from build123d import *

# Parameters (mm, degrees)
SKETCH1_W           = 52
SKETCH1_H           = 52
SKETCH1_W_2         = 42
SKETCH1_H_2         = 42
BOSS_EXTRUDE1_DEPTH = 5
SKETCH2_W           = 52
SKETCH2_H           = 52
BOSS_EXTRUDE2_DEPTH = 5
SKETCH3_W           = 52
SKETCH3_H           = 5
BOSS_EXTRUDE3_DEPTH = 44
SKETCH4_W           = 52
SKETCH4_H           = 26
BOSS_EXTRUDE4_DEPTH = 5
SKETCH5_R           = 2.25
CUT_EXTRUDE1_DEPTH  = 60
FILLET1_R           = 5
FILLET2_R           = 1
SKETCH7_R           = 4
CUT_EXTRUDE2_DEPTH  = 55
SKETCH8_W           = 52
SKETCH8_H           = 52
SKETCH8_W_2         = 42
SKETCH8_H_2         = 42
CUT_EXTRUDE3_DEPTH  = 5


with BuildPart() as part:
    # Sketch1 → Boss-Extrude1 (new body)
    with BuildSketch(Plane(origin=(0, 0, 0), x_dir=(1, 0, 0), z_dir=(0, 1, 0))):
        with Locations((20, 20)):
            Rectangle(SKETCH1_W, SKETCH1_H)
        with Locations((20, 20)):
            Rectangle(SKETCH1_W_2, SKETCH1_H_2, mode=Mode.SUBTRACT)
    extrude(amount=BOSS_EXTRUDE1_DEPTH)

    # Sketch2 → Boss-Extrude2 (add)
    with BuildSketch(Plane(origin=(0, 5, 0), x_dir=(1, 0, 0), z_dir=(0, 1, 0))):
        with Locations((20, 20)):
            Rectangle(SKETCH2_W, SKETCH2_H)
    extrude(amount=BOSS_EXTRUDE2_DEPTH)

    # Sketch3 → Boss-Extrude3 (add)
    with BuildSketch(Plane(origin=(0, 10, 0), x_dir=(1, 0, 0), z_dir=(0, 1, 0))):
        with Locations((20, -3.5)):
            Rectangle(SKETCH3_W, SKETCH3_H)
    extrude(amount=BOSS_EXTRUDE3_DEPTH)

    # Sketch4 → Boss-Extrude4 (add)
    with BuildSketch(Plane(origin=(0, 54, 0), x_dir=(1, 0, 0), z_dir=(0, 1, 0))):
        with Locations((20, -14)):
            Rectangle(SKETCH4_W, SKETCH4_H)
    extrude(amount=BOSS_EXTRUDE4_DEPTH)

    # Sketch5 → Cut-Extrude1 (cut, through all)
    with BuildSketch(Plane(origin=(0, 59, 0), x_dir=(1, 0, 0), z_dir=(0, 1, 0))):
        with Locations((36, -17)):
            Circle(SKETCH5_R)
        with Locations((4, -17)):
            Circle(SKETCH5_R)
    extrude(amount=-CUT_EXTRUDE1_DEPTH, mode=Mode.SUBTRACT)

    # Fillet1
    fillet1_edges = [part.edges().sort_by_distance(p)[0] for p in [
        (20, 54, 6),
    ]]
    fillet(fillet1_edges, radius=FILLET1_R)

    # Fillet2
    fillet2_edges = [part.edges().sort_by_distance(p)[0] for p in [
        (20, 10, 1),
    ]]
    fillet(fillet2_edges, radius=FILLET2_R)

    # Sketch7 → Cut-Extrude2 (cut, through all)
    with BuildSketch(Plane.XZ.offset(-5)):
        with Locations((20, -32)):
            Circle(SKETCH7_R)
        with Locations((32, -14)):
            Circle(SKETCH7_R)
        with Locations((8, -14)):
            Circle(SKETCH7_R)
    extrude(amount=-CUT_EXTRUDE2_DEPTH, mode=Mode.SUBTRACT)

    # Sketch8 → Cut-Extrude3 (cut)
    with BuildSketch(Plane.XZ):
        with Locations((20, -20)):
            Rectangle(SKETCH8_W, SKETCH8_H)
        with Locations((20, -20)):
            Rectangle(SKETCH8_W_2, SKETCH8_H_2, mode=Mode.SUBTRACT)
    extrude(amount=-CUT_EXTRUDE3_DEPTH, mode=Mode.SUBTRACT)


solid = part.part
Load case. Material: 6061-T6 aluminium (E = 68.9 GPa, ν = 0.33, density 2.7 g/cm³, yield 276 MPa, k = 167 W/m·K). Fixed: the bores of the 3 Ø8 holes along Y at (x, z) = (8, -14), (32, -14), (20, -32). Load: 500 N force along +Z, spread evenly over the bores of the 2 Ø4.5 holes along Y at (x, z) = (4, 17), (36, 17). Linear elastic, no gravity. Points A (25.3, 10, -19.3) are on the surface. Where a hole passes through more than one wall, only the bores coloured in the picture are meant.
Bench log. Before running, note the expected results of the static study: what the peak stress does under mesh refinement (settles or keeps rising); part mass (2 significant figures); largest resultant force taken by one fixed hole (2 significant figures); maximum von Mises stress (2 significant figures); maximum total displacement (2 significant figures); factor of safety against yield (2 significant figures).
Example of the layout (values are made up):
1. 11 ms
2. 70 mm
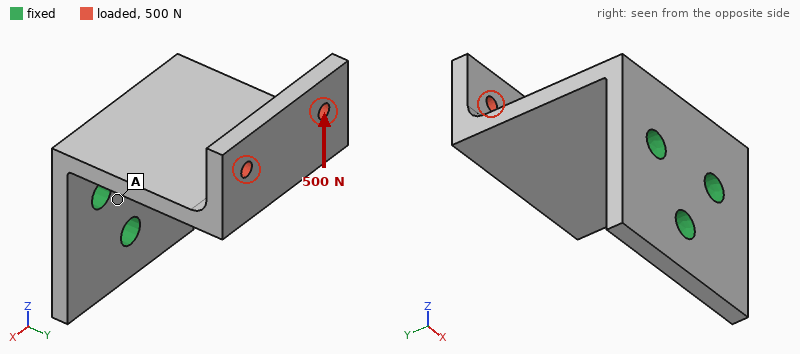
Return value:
1. settles
2. 84 g
3. 270 N
4. 220 MPa
5. 1.1 mm
6. 1.3
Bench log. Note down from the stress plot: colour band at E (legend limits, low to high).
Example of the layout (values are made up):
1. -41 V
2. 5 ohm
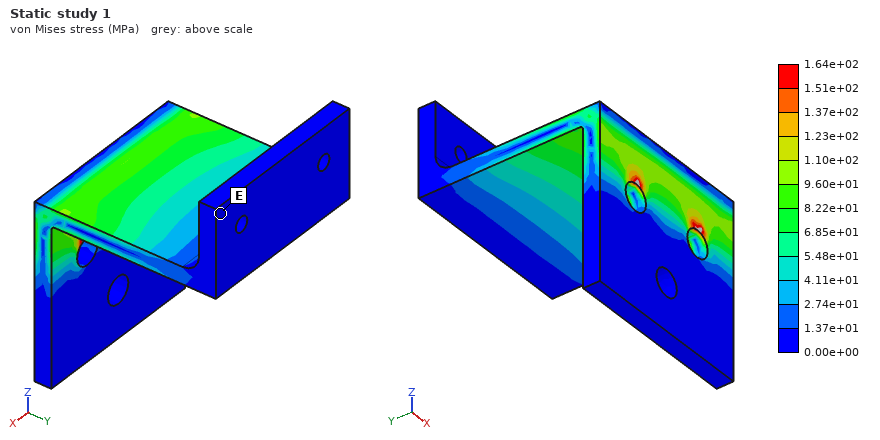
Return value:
1. 0.00e+00 to 1.37e+01 MPa
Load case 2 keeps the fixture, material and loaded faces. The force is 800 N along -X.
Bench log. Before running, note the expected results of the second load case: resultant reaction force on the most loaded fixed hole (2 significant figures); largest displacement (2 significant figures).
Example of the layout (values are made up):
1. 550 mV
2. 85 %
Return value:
1. 1.5 kN
2. 0.26 mm
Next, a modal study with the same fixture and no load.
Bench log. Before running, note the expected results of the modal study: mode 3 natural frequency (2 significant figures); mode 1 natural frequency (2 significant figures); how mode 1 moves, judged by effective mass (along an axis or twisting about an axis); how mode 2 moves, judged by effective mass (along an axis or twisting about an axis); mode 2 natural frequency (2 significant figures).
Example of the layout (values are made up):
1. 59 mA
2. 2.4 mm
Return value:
1. 2200 Hz
2. 690 Hz
3. along Z
4. along X
5. 2000 Hz
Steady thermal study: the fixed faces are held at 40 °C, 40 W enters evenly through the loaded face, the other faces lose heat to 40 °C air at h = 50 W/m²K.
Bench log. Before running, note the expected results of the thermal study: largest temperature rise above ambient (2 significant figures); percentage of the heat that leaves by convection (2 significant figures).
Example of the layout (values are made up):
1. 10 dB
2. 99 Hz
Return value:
1. 54 K
2. 35 %
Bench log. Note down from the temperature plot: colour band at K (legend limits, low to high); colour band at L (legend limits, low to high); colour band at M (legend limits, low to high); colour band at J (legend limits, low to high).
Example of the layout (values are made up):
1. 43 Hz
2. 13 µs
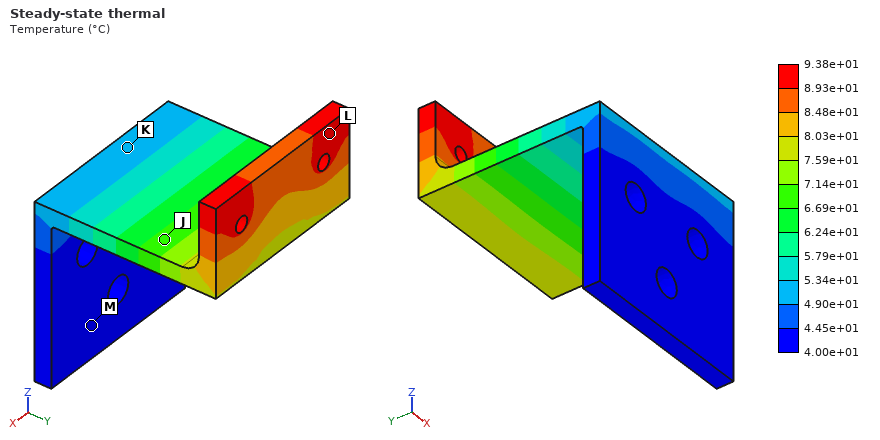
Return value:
1. 4.90e+01 to 5.34e+01 °C
2. 8.93e+01 to 9.38e+01 °C
3. 4.00e+01 to 4.45e+01 °C
4. 6.69e+01 to 7.14e+01 °C
